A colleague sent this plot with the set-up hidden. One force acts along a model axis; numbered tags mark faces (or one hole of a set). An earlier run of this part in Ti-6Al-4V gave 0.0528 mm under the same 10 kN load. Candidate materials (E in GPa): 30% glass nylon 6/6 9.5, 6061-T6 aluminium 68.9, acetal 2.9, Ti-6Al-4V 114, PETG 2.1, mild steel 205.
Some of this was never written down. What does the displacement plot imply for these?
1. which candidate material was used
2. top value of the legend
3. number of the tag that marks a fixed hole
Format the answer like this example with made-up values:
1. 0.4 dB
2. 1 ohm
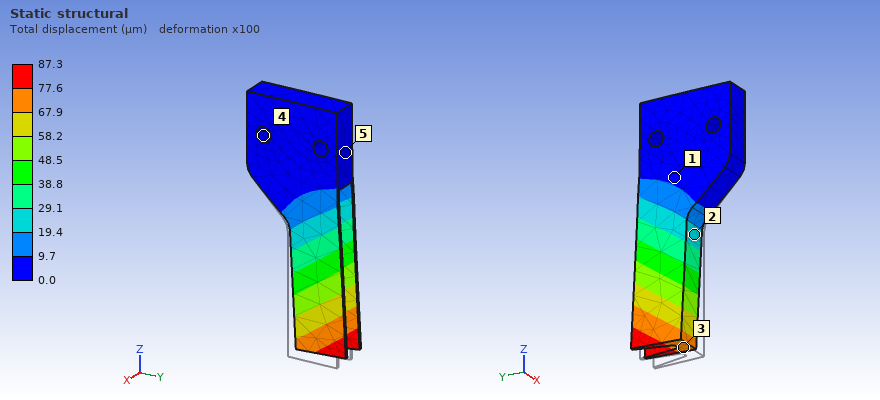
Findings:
1. 6061-T6 aluminium
2. 87.3 µm
3. 4
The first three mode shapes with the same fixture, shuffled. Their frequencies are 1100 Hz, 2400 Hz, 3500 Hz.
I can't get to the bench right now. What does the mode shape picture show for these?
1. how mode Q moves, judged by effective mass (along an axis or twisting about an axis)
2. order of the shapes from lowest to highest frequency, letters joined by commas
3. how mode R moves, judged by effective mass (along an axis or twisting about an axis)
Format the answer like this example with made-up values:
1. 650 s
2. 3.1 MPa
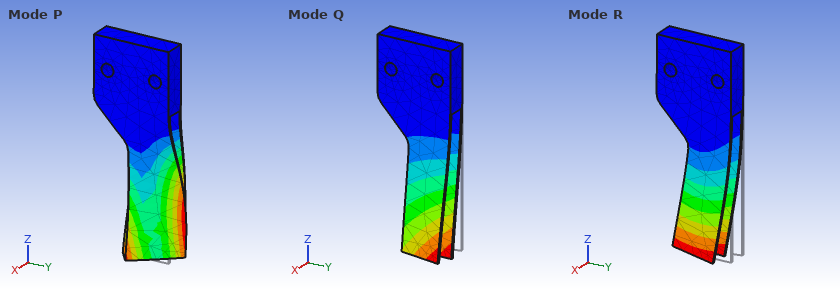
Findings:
1. along X
2. Q, R, P
3. along Y
